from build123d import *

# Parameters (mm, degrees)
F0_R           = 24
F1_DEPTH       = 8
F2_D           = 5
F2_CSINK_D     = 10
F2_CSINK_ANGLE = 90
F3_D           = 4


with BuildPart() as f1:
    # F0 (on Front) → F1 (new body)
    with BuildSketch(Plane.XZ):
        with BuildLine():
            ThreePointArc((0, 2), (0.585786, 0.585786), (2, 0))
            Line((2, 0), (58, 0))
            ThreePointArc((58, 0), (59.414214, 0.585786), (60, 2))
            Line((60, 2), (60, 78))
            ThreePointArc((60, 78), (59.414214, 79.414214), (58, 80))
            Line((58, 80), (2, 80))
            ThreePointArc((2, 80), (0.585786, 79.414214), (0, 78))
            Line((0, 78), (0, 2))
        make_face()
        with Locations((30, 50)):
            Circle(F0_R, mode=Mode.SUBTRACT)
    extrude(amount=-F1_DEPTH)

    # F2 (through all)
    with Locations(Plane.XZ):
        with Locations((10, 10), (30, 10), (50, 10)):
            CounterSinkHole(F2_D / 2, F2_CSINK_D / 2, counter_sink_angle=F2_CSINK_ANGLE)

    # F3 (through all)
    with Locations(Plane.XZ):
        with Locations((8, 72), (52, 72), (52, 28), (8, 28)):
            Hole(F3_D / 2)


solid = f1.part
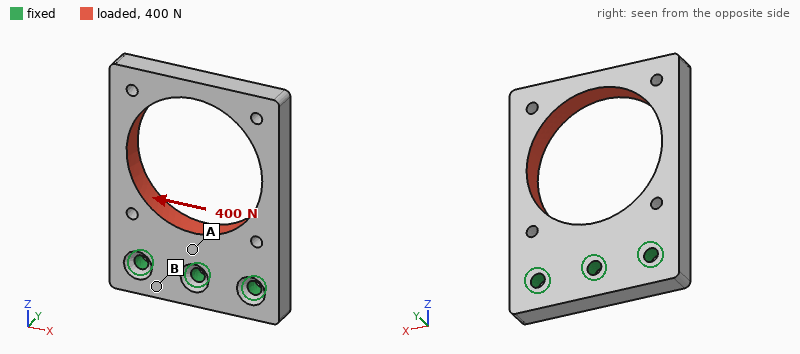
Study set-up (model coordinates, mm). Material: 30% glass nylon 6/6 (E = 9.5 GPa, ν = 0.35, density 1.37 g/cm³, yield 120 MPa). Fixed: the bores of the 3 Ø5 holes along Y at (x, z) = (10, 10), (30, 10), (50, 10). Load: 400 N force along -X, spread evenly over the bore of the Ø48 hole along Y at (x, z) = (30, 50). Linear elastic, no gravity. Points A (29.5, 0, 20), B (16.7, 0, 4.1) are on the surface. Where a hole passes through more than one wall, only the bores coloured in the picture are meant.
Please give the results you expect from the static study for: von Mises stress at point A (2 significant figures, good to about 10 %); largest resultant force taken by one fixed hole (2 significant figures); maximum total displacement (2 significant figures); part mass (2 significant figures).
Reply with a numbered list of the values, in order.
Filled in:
1. 3.8 MPa
2. 370 N
3. 0.22 mm
4. 31 g
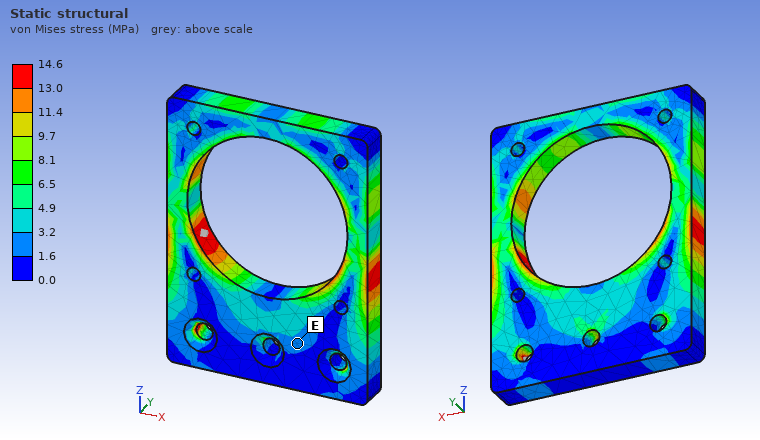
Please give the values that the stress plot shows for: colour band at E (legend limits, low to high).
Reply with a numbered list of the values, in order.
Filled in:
1. 1.6 to 3.2 MPa
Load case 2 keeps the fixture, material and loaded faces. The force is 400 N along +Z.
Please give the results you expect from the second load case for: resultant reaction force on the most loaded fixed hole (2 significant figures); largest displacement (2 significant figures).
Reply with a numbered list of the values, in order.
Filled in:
1. 200 N
2. 48 µm
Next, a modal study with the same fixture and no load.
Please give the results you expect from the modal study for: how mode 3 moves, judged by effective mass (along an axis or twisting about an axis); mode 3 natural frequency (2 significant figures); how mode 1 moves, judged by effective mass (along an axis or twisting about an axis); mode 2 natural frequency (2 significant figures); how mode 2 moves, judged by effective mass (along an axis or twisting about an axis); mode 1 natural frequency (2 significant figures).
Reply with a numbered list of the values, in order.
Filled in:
1. along X
2. 1700 Hz
3. along Y
4. 1300 Hz
5. twisting about Z
6. 590 Hz
